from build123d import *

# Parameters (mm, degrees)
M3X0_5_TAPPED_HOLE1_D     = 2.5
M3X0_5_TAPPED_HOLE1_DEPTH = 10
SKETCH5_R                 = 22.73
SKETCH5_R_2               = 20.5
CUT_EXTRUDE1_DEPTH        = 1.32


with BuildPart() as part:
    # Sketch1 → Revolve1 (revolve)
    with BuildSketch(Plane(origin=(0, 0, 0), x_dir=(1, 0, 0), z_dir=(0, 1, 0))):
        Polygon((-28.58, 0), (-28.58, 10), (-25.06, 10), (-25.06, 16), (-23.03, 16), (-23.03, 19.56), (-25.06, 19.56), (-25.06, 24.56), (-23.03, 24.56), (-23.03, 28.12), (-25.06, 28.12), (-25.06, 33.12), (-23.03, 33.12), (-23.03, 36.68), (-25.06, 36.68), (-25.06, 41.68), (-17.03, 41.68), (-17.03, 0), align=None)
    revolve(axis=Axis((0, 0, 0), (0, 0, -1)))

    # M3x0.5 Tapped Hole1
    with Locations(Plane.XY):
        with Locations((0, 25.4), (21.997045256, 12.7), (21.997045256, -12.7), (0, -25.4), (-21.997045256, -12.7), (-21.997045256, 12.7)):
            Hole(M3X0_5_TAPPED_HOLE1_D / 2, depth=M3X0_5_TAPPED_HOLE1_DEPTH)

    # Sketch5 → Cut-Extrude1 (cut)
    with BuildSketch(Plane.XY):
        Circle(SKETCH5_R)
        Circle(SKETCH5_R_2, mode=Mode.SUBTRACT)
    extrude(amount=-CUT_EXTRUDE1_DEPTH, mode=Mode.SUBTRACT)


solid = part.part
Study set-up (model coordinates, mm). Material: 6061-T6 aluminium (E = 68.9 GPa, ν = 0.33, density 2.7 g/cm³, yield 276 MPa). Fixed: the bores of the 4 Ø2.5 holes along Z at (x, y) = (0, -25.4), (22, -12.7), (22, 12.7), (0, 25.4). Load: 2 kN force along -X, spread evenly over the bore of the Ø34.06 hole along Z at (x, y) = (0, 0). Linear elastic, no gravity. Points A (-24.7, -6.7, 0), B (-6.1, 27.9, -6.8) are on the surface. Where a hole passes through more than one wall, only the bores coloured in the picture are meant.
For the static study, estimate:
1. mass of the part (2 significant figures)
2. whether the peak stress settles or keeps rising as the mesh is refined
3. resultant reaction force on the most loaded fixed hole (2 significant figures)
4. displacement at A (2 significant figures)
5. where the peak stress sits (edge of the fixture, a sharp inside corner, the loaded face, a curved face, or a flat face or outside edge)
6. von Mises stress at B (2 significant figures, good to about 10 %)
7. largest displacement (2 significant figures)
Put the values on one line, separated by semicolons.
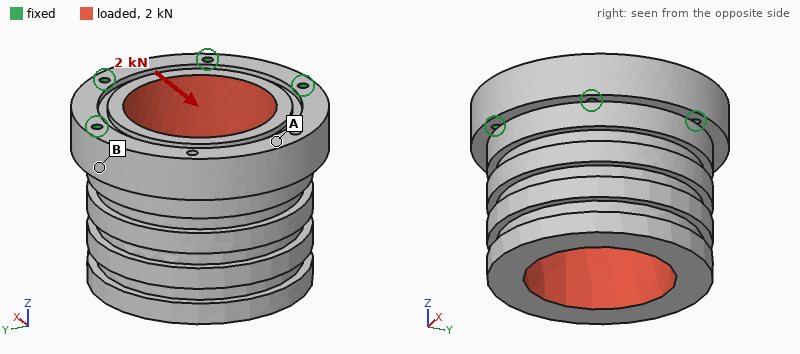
120 g; keeps rising; 740 N; 8.8 µm; edge of the fixture; 6.0 MPa; 16 µm
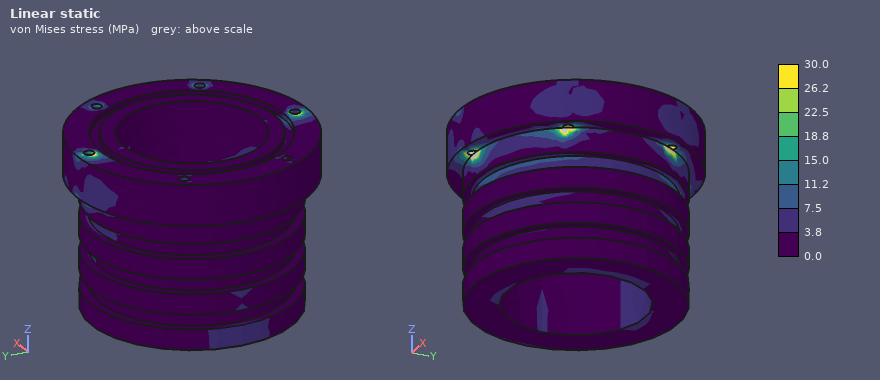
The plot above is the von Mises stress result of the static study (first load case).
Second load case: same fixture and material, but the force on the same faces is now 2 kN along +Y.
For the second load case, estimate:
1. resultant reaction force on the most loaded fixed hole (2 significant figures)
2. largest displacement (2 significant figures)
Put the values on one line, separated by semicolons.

870 N; 5.6 µm
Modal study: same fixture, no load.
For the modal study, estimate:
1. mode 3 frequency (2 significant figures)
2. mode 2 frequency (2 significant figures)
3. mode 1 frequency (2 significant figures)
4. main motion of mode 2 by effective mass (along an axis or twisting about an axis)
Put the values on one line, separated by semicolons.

13 kHz; 10 kHz; 5900 Hz; along Y
